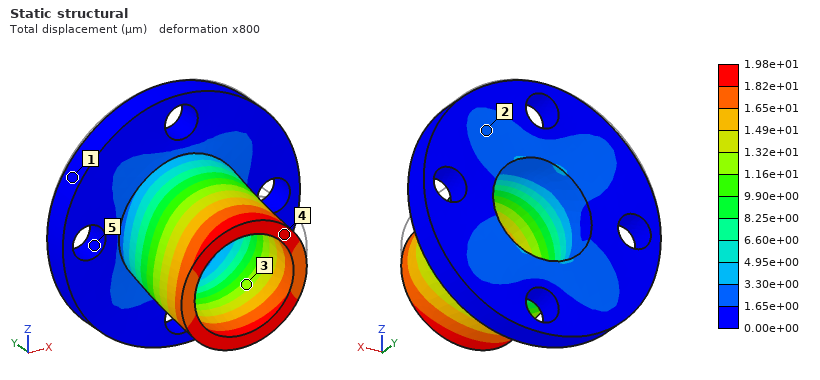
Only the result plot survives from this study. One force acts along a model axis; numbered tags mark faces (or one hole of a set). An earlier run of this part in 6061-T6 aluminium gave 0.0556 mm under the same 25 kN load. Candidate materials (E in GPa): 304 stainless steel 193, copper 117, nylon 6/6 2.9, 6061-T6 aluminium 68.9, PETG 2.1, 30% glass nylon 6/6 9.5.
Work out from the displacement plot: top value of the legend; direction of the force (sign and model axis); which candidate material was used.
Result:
1.98e+01 µm
-Z
304 stainless steel
